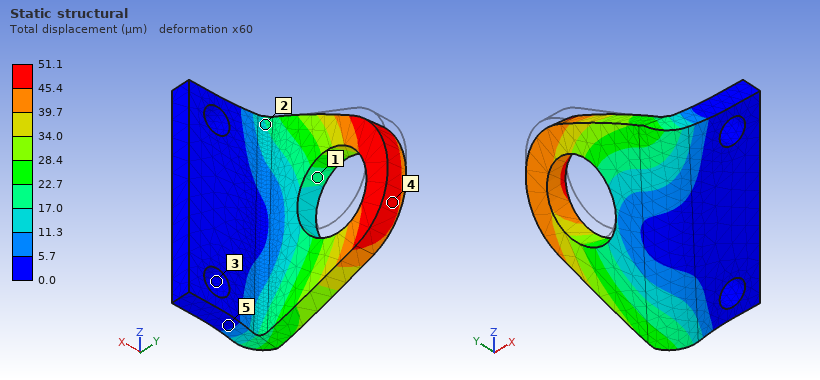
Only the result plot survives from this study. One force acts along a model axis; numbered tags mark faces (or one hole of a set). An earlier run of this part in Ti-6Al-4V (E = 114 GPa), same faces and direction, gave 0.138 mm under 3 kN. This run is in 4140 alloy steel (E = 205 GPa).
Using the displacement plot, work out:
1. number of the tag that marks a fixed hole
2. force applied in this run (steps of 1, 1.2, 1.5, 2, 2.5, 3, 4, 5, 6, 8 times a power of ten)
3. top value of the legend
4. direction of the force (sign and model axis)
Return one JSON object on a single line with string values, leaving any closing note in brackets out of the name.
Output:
{"number of the tag that marks a fixed hole": "3", "force applied in this run": "2 kN", "top value of the legend": "51.1 µm", "direction of the force": "-Z"}
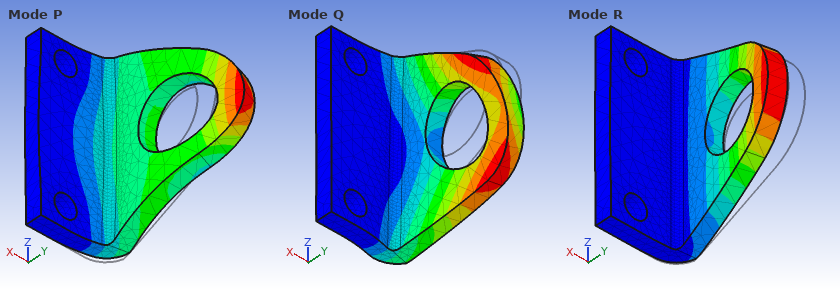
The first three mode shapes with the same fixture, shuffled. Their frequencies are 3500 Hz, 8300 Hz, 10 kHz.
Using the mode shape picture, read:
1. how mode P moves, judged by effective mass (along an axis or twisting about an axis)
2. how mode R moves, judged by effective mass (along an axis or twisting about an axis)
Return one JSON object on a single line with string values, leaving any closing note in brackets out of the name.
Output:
{"how mode P moves, judged by effective mass": "along Y", "how mode R moves, judged by effective mass": "along X"}
